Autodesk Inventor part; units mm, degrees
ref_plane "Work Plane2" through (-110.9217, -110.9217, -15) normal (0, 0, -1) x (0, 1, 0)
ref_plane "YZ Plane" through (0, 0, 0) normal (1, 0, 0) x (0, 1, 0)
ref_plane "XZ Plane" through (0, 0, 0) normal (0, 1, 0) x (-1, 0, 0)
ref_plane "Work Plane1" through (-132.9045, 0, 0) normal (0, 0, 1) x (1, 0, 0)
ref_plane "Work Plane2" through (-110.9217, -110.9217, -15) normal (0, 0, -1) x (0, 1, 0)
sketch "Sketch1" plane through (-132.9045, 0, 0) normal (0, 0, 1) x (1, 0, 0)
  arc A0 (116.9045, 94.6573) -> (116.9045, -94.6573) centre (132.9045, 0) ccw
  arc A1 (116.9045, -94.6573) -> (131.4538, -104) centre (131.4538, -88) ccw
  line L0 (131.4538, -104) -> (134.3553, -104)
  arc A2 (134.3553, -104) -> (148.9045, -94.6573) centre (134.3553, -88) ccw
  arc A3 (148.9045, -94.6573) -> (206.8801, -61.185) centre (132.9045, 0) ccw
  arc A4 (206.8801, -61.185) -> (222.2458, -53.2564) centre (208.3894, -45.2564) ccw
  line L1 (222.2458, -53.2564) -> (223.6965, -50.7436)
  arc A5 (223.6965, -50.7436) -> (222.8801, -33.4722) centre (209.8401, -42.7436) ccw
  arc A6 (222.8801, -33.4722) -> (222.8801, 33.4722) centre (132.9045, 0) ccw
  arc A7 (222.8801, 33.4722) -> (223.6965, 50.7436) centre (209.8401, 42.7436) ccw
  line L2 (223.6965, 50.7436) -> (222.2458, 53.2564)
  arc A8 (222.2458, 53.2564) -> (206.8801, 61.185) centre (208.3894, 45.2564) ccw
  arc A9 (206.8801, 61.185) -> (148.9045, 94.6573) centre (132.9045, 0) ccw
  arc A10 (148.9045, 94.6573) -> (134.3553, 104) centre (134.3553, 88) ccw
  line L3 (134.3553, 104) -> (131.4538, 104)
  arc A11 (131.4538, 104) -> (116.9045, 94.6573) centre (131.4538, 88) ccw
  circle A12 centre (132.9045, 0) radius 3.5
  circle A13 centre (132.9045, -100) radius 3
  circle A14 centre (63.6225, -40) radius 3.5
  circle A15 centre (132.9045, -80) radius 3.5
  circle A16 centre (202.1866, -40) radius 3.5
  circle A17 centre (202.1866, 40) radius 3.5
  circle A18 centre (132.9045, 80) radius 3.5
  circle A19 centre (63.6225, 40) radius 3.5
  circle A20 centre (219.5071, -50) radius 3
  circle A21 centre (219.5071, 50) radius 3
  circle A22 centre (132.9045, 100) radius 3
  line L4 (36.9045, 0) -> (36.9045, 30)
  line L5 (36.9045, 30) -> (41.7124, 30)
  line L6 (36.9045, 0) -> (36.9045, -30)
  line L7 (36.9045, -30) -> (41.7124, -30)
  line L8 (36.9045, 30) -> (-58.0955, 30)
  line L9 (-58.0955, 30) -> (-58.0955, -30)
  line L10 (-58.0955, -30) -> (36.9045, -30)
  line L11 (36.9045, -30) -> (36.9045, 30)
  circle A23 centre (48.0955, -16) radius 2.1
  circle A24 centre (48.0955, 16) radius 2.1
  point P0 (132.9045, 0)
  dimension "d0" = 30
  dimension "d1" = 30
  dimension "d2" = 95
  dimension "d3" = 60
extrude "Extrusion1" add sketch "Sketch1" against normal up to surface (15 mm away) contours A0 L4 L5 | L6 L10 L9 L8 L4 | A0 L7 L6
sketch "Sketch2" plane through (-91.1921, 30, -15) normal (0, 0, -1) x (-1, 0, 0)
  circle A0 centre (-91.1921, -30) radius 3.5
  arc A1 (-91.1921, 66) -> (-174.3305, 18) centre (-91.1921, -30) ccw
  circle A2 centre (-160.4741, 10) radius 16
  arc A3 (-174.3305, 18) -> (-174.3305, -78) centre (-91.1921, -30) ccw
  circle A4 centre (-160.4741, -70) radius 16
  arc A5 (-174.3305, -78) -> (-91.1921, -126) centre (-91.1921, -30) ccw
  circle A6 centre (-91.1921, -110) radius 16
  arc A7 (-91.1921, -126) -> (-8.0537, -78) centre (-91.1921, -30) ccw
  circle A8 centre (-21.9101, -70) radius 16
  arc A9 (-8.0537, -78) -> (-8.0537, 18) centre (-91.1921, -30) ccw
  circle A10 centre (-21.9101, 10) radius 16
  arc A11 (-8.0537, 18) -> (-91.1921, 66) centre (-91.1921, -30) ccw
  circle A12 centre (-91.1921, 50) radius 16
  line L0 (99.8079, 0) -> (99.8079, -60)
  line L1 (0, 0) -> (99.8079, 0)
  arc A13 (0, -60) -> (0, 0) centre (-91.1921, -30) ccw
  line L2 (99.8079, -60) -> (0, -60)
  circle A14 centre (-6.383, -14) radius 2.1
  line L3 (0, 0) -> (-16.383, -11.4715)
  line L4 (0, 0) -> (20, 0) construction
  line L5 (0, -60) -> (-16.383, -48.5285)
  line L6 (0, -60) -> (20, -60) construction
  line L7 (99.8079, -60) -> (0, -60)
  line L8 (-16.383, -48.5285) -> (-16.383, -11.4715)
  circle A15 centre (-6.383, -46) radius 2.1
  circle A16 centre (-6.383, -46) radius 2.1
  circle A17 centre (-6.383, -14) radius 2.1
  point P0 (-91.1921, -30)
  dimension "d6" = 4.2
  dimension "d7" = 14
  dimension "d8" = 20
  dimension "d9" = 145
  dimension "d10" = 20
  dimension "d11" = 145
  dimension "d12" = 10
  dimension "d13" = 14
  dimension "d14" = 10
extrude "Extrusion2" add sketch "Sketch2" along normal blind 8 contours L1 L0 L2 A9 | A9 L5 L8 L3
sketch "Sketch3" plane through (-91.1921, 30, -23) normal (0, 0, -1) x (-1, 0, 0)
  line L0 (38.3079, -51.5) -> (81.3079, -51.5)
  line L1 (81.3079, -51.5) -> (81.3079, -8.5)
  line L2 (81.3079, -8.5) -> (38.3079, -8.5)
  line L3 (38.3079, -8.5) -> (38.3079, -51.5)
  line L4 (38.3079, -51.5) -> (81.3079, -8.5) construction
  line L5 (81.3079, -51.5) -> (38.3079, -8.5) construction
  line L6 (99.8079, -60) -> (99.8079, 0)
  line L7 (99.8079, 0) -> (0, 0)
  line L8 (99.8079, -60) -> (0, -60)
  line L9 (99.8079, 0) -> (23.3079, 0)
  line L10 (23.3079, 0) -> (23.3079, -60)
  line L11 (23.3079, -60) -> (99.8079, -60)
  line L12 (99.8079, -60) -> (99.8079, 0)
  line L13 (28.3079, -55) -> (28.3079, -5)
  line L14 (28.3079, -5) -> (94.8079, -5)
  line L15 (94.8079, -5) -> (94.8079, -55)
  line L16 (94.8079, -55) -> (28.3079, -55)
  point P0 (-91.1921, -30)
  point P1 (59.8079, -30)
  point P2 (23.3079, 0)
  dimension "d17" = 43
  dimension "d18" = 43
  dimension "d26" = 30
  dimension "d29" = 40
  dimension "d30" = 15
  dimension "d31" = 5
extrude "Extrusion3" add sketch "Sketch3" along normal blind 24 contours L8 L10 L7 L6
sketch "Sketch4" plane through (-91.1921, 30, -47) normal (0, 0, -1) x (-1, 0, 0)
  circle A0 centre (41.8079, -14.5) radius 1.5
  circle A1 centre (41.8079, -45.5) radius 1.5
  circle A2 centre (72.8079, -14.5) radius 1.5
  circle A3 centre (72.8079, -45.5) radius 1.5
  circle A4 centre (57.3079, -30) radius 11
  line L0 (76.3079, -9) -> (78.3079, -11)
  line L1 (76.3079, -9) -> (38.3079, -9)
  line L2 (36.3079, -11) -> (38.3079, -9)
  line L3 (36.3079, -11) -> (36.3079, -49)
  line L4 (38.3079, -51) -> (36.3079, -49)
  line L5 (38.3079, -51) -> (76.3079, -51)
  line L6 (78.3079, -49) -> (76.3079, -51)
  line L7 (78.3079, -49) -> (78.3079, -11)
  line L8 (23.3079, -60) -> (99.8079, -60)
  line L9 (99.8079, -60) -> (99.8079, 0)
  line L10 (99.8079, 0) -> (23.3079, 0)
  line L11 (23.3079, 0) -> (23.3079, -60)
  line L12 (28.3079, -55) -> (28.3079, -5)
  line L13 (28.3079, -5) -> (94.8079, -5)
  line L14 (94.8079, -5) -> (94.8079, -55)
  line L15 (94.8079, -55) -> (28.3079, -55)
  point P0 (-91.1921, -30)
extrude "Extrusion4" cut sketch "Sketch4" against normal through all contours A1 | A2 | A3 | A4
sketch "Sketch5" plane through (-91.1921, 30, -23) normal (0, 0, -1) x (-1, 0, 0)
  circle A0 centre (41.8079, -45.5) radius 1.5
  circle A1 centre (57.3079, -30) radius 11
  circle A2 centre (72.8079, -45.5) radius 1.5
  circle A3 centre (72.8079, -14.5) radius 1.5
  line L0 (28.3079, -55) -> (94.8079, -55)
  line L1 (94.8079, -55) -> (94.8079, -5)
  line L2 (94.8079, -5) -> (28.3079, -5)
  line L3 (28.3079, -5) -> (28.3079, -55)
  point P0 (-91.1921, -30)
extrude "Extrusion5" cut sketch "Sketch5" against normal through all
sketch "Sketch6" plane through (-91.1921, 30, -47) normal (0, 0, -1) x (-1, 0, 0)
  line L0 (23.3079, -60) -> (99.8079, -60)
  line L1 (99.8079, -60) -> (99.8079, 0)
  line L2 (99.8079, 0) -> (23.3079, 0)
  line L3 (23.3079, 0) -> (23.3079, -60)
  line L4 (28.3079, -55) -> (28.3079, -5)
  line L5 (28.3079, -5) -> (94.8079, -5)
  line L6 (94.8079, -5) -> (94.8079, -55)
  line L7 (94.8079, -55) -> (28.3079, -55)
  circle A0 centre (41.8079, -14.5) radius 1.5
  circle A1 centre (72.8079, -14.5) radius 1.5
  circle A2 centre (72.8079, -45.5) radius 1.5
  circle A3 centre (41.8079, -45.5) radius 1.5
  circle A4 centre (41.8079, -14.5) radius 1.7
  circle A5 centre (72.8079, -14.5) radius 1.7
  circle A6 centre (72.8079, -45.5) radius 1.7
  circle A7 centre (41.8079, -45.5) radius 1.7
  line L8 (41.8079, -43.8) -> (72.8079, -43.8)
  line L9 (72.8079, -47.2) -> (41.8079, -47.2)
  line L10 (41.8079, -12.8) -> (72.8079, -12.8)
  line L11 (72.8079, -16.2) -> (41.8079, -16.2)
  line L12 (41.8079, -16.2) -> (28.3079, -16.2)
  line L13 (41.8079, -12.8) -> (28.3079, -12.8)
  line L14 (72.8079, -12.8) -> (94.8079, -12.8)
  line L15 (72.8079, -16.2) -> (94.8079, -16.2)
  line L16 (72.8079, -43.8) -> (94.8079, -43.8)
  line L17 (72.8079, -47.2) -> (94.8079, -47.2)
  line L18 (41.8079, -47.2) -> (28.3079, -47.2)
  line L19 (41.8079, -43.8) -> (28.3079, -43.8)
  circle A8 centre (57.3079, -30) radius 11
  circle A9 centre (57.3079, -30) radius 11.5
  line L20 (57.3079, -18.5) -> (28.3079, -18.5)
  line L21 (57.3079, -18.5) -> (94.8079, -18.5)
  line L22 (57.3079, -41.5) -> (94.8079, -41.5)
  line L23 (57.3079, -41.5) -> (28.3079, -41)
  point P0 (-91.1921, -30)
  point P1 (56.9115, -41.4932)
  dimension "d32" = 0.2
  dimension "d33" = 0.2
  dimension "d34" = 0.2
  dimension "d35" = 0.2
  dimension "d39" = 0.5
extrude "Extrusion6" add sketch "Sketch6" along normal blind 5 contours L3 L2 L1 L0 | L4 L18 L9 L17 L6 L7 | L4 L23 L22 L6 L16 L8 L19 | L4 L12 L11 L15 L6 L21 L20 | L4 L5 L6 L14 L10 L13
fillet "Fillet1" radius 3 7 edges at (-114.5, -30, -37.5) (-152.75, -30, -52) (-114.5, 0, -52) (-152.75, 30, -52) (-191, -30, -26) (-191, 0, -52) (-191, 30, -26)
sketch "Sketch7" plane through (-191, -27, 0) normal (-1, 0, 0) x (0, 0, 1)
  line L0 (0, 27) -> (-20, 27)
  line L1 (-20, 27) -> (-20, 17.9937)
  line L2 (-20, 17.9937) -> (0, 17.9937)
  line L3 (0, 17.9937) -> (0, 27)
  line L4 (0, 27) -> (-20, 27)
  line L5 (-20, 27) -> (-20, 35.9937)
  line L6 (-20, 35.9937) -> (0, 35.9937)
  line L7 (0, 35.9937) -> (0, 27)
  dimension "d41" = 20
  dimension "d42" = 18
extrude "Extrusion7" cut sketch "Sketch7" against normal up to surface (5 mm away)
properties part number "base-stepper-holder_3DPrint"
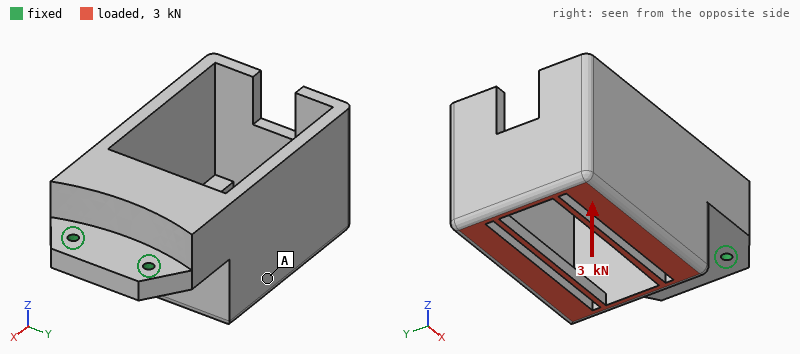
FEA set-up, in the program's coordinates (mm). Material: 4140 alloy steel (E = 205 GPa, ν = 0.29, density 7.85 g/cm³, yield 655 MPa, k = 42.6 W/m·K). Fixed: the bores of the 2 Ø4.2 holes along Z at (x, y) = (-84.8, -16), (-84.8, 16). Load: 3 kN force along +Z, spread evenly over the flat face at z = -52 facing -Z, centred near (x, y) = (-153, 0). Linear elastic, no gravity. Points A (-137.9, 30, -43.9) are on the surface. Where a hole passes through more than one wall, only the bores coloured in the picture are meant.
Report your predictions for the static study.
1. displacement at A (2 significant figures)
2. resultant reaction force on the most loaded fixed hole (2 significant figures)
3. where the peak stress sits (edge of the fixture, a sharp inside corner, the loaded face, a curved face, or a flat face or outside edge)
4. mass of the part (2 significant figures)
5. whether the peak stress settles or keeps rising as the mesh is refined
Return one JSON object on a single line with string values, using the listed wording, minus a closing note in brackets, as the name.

{"displacement at A": "0.36 mm", "resultant reaction force on the most loaded fixed hole": "1.5 kN", "where the peak stress sits": "edge of the fixture", "mass of the part": "830 g", "whether the peak stress settles or keeps rising as the mesh is refined": "keeps rising"}
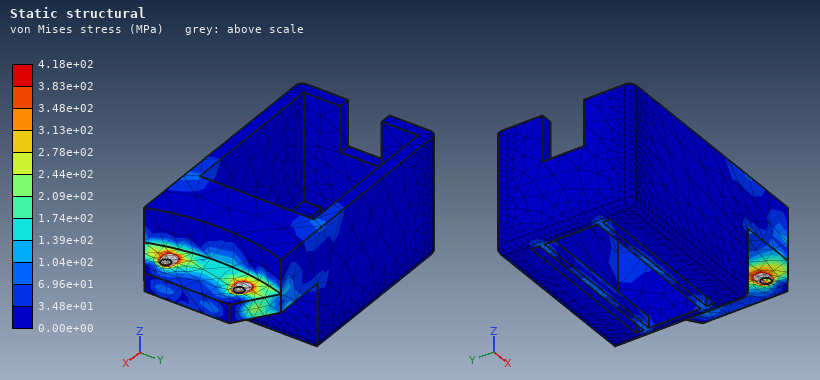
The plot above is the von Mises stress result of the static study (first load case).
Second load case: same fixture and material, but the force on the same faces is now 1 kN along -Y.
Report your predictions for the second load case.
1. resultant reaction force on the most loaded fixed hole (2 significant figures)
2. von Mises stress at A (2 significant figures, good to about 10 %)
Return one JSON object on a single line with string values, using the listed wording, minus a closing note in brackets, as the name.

{"resultant reaction force on the most loaded fixed hole": "2.2 kN", "von Mises stress at A": "8.3 MPa"}
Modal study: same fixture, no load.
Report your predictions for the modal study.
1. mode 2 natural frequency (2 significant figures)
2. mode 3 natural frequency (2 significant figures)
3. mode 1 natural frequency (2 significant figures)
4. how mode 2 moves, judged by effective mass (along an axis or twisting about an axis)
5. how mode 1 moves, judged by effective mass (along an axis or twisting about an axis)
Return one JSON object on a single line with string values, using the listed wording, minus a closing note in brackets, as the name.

{"mode 2 natural frequency": "850 Hz", "mode 3 natural frequency": "1700 Hz", "mode 1 natural frequency": "500 Hz", "how mode 2 moves, judged by effective mass": "along Y", "how mode 1 moves, judged by effective mass": "along Z"}
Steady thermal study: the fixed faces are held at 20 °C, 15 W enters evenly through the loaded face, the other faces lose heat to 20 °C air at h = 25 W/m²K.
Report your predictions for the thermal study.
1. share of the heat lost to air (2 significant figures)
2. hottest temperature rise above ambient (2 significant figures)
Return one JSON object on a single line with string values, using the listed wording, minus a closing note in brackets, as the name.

{"share of the heat lost to air": "68 %", "hottest temperature rise above ambient": "29 K"}
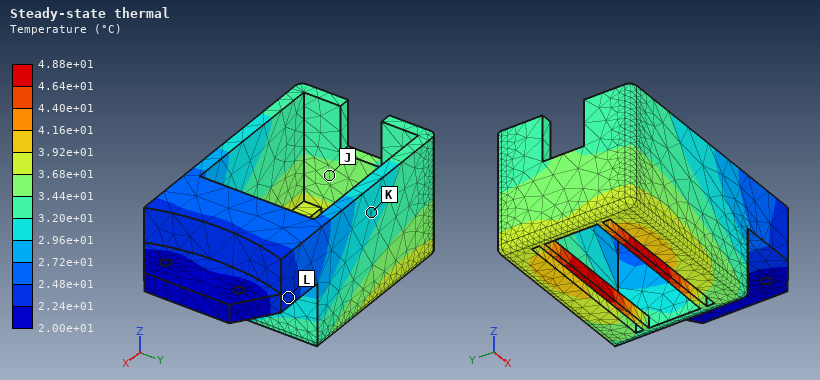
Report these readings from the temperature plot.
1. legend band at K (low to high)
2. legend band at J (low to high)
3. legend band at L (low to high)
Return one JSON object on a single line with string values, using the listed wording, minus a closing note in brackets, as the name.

{"legend band at K": "2.96e+01 to 3.20e+01 °C", "legend band at J": "3.44e+01 to 3.68e+01 °C", "legend band at L": "2.24e+01 to 2.48e+01 °C"}
